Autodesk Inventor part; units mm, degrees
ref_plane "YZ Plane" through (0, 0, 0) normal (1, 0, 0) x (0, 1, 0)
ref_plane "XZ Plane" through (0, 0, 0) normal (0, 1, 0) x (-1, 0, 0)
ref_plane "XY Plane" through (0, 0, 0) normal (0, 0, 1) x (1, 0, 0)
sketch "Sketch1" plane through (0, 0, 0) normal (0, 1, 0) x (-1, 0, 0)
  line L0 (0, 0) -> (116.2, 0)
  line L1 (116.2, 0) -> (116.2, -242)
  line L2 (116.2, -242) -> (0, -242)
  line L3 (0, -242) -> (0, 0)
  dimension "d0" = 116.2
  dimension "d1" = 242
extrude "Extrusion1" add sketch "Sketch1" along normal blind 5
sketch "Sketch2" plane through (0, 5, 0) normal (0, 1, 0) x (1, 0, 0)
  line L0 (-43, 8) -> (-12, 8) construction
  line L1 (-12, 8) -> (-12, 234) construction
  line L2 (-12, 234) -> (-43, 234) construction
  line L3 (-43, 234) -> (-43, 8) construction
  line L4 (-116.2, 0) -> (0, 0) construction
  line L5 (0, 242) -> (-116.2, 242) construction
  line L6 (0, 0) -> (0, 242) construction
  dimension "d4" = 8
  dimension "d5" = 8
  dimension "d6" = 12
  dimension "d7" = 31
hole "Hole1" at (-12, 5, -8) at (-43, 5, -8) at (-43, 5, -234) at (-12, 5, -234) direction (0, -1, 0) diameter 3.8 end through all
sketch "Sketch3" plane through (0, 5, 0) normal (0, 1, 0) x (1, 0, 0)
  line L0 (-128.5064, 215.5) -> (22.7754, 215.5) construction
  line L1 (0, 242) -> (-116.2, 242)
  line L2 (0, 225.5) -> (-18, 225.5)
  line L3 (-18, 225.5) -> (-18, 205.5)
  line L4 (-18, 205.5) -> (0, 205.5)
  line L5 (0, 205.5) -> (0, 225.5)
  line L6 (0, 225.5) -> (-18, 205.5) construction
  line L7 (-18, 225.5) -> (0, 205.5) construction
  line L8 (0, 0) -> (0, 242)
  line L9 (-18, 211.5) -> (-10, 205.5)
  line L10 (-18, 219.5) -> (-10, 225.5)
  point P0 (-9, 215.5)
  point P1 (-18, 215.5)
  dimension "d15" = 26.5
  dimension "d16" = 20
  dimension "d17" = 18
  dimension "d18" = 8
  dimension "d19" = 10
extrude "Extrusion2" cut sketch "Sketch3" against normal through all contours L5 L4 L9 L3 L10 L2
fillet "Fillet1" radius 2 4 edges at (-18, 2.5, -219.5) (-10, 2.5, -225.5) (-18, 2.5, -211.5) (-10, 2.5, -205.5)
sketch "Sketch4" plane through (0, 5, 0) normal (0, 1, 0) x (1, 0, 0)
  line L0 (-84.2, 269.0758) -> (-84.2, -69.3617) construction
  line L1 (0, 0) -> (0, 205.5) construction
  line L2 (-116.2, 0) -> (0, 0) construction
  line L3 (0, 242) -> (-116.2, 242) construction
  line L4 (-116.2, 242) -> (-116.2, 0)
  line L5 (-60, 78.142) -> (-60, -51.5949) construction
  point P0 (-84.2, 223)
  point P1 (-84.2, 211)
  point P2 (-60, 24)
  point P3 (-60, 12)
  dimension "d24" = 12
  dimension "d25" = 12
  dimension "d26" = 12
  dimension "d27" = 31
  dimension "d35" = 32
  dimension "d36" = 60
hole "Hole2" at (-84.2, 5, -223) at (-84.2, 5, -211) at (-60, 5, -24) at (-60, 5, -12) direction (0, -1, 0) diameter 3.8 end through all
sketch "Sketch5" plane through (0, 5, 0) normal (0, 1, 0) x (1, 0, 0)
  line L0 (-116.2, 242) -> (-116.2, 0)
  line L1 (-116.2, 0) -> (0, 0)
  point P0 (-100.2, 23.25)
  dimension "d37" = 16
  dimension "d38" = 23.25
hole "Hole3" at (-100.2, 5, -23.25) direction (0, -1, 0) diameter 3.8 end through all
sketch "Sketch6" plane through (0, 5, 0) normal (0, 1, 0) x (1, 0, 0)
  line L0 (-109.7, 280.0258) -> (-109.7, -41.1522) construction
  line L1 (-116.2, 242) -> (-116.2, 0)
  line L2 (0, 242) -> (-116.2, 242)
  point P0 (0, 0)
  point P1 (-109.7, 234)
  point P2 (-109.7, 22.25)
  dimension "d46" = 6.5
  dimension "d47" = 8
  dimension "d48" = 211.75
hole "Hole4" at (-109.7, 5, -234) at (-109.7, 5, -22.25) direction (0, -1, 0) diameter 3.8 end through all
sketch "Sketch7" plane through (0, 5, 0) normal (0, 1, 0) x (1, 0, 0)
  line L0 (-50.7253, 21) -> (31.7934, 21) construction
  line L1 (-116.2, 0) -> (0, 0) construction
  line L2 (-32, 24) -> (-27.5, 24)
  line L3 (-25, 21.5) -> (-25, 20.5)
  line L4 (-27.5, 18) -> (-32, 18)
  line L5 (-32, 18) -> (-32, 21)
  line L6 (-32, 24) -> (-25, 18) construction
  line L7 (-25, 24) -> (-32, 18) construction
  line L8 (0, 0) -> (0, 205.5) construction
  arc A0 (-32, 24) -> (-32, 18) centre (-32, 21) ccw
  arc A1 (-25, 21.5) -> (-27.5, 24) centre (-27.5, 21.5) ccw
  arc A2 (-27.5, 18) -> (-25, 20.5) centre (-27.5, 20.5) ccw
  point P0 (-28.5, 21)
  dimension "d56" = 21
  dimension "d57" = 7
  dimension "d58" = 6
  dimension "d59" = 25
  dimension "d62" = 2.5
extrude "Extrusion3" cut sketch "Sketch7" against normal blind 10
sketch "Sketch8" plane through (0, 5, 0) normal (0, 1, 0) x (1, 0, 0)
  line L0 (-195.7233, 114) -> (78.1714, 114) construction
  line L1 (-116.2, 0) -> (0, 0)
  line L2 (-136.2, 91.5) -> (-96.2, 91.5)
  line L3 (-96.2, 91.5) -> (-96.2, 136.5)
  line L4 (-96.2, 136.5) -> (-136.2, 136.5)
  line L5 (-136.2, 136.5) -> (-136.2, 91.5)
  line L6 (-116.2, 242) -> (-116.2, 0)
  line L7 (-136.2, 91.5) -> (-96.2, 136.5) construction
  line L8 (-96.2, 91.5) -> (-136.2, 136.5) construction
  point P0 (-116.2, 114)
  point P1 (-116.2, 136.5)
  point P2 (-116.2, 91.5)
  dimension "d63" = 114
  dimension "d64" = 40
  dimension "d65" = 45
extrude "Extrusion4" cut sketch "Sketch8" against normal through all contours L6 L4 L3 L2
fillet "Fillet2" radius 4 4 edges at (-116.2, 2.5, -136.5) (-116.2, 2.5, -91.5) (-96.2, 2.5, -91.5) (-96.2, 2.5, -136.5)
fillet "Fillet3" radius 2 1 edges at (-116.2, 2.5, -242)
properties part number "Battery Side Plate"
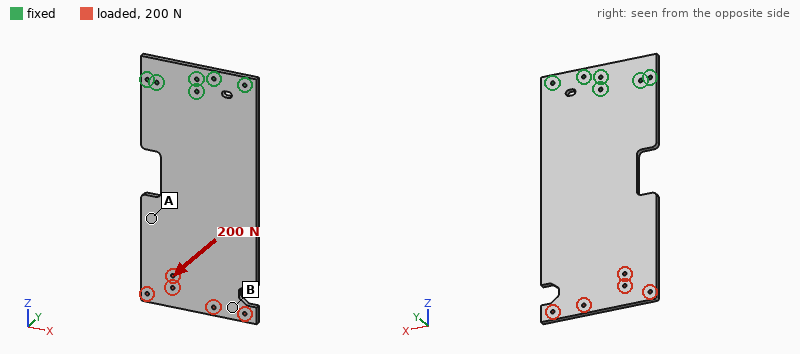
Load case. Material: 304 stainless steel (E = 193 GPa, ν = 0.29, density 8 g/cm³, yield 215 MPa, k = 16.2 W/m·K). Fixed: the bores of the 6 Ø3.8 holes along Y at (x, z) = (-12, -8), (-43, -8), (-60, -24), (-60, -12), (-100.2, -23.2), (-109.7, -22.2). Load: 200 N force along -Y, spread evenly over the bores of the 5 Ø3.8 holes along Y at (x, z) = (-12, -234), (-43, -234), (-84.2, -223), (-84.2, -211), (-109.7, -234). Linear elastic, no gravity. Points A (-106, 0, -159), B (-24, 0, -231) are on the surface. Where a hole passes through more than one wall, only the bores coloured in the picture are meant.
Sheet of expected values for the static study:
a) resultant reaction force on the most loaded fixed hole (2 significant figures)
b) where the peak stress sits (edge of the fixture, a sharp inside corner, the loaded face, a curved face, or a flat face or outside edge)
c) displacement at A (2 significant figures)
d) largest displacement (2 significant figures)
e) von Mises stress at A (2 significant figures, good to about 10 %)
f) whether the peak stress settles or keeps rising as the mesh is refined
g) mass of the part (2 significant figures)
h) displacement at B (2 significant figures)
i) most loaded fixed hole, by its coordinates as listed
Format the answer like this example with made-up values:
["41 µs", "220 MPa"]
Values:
["1.2 kN", "edge of the fixture", "1.4 mm", "3.0 mm", "21 MPa", "keeps rising", "1.1 kg", "2.7 mm", "(-60, -24)"]
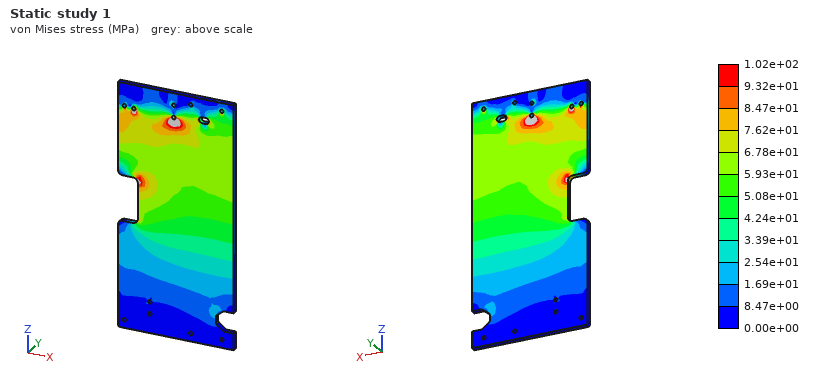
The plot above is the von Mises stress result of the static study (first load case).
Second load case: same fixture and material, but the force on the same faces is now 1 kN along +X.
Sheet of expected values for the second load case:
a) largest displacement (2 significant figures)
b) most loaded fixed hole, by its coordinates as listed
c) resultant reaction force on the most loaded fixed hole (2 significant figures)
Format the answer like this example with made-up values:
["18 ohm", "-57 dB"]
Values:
["47 µm", "(-12, -8)", "1.8 kN"]
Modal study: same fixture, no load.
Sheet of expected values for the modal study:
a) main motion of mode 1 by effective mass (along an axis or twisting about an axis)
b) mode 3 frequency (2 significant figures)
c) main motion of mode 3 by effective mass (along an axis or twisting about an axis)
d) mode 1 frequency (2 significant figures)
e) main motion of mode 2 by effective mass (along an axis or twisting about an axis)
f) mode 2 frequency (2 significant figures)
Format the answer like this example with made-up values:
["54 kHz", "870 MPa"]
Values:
["along Y", "500 Hz", "along Y", "81 Hz", "twisting about Z", "320 Hz"]
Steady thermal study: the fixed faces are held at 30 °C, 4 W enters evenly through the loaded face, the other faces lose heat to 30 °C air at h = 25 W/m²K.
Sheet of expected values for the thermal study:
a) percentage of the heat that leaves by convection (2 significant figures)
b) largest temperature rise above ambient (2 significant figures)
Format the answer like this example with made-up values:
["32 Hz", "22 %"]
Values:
["99 %", "17 K"]
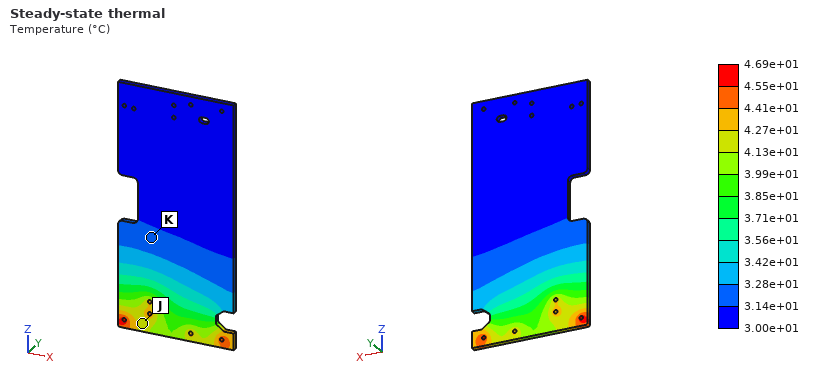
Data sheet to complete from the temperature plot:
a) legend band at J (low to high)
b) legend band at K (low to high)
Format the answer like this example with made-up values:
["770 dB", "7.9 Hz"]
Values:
["4.13e+01 to 4.27e+01 °C", "3.14e+01 to 3.28e+01 °C"]
